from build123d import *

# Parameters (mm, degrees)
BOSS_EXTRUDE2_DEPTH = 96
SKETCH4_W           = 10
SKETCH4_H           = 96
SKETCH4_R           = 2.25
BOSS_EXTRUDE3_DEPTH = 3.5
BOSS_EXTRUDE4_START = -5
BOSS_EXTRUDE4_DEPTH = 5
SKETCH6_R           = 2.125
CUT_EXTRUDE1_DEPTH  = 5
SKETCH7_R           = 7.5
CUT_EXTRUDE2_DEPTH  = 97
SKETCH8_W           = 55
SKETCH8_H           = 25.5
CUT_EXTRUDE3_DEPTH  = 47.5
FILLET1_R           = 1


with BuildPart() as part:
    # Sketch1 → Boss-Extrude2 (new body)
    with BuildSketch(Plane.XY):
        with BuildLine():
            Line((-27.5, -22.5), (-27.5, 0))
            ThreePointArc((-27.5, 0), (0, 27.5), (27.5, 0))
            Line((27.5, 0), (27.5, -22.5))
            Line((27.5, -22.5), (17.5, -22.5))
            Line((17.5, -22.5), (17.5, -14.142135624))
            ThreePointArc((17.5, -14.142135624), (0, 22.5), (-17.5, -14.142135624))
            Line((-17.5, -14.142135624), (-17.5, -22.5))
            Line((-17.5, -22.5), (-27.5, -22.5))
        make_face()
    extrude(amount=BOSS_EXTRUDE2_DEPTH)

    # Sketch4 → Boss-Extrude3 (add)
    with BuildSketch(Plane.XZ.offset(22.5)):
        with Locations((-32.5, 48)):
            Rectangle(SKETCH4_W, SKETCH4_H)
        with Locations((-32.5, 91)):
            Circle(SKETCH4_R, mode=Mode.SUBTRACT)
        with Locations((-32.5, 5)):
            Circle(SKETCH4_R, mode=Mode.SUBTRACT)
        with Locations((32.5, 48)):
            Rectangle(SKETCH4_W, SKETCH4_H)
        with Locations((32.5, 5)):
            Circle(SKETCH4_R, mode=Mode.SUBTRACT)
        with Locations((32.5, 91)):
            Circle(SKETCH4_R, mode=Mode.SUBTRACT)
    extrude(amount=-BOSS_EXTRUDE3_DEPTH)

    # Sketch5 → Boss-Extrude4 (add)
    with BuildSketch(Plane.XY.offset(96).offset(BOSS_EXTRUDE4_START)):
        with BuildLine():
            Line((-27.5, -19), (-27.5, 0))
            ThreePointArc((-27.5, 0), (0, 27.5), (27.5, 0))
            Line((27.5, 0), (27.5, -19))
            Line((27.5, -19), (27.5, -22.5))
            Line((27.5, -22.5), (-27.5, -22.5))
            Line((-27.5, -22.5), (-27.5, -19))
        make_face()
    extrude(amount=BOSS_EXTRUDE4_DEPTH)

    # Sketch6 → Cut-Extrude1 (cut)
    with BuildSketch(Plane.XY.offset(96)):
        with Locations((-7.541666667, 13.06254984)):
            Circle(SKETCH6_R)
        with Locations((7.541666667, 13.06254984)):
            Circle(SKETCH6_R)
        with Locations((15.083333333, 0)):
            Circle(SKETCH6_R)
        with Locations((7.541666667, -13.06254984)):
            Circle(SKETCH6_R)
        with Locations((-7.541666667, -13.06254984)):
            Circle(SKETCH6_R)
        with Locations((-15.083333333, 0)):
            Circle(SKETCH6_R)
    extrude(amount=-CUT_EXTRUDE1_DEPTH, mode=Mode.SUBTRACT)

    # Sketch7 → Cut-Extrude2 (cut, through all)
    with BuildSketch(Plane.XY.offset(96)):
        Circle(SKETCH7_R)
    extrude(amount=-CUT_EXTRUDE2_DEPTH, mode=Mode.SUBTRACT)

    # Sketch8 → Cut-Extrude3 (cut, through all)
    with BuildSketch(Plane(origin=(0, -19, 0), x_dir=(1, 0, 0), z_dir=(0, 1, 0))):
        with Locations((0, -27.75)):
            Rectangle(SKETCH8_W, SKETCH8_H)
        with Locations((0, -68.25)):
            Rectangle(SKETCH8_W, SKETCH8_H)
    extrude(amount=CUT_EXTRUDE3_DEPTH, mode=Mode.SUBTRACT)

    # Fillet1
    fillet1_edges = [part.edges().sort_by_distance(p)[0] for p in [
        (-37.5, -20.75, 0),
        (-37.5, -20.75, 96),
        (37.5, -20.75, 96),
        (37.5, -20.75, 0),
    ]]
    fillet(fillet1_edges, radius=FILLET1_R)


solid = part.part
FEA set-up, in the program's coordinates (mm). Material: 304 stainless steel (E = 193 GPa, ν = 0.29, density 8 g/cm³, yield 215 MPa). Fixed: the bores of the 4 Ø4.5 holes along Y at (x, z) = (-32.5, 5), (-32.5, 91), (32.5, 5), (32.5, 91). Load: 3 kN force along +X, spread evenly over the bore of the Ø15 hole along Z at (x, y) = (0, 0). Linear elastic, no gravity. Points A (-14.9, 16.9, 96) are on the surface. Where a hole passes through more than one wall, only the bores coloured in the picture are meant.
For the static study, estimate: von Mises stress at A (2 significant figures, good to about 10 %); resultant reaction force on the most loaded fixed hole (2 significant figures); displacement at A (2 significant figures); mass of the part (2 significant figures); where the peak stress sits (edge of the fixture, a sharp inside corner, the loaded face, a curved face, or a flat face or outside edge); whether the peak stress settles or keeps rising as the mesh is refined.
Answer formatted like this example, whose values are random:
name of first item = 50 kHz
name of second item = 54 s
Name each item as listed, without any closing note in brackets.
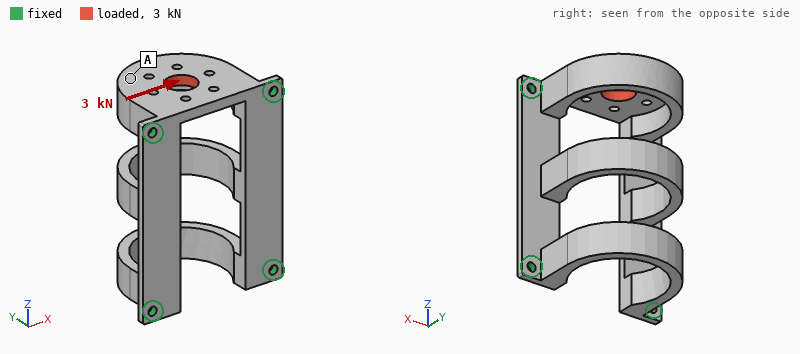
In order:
von Mises stress at A = 7.9 MPa
resultant reaction force on the most loaded fixed hole = 1.8 kN
displacement at A = 12 µm
mass of the part = 410 g
where the peak stress sits = edge of the fixture
whether the peak stress settles or keeps rising as the mesh is refined = keeps rising
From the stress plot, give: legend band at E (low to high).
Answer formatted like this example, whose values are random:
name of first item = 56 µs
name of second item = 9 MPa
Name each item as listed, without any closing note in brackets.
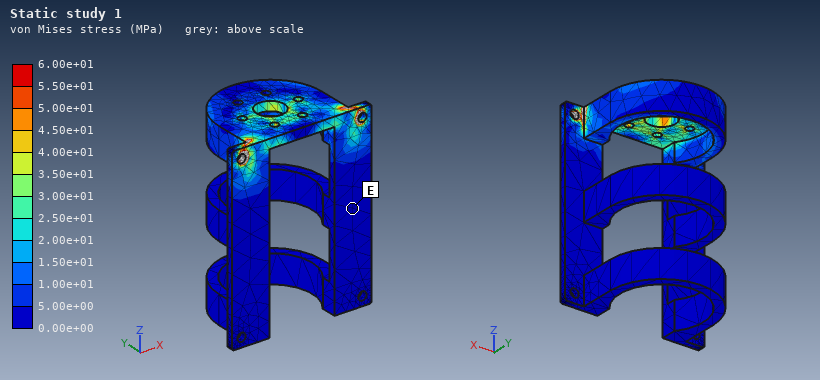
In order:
legend band at E = 0.00e+00 to 5.00e+00 MPa
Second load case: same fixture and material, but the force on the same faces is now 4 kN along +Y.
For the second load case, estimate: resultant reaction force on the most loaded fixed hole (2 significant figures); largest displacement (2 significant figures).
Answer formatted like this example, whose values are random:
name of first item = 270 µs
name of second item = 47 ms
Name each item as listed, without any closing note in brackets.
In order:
resultant reaction force on the most loaded fixed hole = 2.3 kN
largest displacement = 82 µm
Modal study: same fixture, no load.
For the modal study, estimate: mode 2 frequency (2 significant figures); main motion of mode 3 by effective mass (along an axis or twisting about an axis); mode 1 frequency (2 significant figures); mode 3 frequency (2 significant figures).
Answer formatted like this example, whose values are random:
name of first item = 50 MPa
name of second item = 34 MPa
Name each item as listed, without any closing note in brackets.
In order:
mode 2 frequency = 1400 Hz
main motion of mode 3 by effective mass = along X
mode 1 frequency = 1200 Hz
mode 3 frequency = 1500 Hz
